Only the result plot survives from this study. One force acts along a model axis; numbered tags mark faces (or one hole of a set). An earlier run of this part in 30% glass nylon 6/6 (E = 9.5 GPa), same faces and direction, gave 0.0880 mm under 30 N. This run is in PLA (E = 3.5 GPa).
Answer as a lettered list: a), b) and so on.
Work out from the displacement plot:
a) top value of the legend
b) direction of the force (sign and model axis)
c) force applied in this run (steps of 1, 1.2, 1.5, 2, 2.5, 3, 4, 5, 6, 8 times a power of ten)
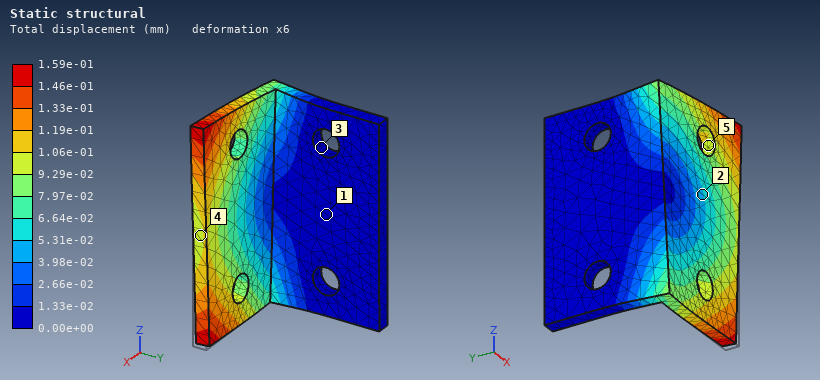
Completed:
a) 1.59e-01 mm
b) +Z
c) 20 N
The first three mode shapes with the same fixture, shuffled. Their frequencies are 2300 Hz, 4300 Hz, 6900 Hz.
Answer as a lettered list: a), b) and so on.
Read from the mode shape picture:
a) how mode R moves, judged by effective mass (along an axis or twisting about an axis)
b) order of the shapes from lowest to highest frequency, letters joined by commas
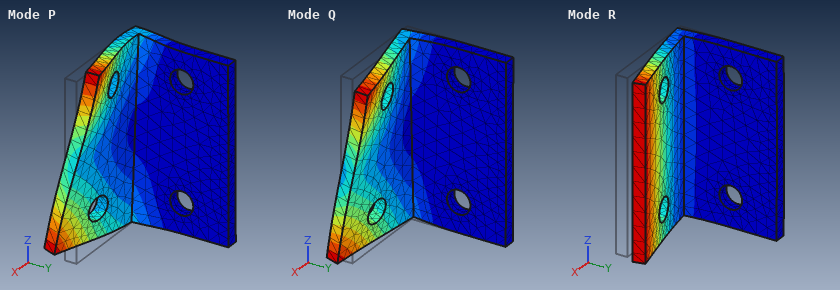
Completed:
a) along Y
b) R, Q, P
